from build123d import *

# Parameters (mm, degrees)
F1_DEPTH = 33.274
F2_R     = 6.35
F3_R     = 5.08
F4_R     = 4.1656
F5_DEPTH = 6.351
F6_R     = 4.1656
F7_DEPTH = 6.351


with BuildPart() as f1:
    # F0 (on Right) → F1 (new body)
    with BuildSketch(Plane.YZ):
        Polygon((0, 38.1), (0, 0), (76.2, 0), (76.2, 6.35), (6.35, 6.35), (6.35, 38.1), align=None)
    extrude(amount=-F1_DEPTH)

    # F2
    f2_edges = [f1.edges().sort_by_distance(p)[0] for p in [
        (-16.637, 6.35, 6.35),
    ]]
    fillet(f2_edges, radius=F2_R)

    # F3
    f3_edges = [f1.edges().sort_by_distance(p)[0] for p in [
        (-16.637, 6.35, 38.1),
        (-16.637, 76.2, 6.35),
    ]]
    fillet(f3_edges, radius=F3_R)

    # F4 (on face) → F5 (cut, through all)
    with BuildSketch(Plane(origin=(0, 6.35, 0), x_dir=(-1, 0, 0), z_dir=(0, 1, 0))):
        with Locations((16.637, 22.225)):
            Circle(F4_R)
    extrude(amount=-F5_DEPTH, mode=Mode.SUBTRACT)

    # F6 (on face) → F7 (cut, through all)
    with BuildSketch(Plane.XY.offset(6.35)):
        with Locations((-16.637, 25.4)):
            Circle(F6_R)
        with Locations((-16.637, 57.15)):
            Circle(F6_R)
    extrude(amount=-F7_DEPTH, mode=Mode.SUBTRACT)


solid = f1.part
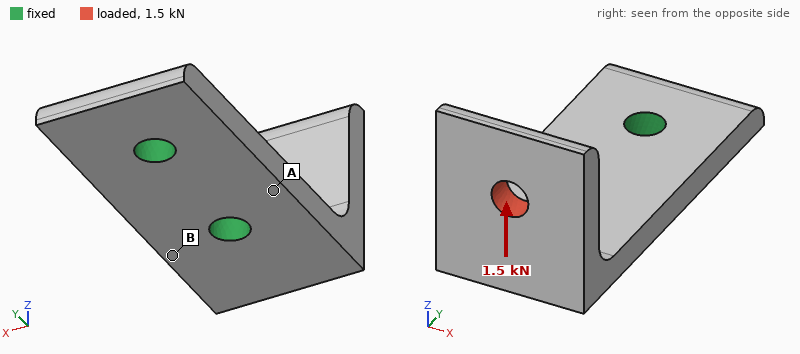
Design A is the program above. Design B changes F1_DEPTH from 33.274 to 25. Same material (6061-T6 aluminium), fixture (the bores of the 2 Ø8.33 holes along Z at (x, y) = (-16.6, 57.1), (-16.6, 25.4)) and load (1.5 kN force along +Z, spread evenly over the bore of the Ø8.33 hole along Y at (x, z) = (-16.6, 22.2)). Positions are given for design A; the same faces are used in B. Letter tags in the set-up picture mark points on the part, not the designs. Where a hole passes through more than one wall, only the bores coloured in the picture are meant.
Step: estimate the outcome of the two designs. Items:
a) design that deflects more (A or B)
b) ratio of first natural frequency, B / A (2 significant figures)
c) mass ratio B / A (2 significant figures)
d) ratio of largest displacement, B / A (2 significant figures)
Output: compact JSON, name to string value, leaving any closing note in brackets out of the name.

{"design that deflects more": "B", "ratio of first natural frequency, B / A": "1.0", "mass ratio B / A": "0.74", "ratio of largest displacement, B / A": "1.3"}
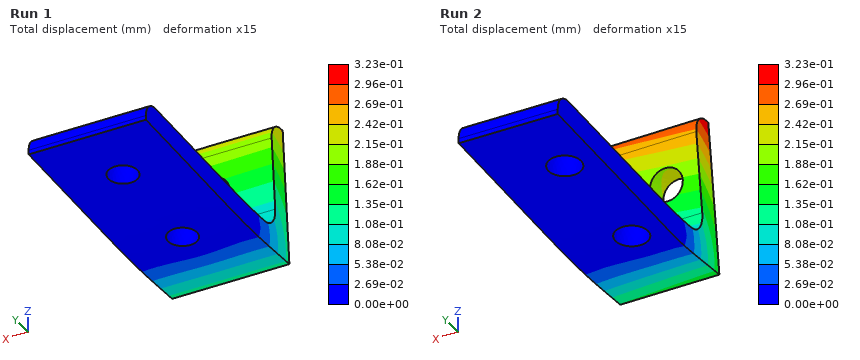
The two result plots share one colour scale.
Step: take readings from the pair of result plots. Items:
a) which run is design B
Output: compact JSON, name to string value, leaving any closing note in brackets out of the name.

{"which run is design B": "Run 2"}
